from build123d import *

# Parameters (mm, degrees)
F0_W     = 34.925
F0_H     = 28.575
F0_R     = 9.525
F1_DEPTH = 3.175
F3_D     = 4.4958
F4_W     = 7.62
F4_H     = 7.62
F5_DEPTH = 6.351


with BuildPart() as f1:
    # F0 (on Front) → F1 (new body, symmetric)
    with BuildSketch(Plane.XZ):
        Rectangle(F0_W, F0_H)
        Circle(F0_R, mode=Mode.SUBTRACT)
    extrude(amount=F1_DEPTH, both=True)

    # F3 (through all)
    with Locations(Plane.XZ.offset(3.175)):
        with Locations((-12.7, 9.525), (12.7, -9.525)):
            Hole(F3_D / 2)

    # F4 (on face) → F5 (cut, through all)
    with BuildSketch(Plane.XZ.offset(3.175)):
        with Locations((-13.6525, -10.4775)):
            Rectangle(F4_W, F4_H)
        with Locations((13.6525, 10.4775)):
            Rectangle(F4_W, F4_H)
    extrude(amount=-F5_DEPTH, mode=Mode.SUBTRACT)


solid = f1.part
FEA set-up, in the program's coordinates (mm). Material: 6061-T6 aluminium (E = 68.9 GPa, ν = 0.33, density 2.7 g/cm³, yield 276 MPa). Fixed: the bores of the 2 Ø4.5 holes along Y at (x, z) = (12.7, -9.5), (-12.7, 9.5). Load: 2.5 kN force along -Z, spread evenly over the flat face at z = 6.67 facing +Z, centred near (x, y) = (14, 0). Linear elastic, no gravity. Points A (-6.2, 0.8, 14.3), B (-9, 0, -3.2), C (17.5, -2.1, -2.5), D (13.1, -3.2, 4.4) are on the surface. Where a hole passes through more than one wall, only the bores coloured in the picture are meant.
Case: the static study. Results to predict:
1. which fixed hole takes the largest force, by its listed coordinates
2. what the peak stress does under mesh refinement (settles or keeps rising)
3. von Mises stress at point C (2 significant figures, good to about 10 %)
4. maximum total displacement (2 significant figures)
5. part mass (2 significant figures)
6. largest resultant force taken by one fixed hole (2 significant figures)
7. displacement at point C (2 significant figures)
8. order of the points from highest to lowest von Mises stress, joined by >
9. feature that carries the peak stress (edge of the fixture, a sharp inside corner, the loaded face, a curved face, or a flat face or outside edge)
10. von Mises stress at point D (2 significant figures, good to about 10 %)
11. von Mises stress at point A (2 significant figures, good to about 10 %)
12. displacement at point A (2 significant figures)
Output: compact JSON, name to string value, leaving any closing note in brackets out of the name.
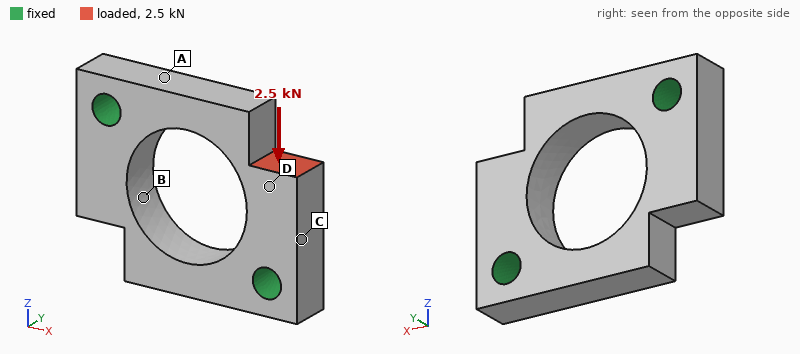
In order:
{"which fixed hole takes the largest force, by its listed coordinates": "(12.7, -9.5)", "what the peak stress does under mesh refinement": "keeps rising", "von Mises stress at point C": "42 MPa", "maximum total displacement": "11 µm", "part mass": "9.7 g", "largest resultant force taken by one fixed hole": "2.4 kN", "displacement at point C": "4.9 µm", "order of the points from highest to lowest von Mises stress, joined by >": "D > C > A > B", "feature that carries the peak stress": "edge of the fixture", "von Mises stress at point D": "54 MPa", "von Mises stress at point A": "14 MPa", "displacement at point A": "1.9 µm"}
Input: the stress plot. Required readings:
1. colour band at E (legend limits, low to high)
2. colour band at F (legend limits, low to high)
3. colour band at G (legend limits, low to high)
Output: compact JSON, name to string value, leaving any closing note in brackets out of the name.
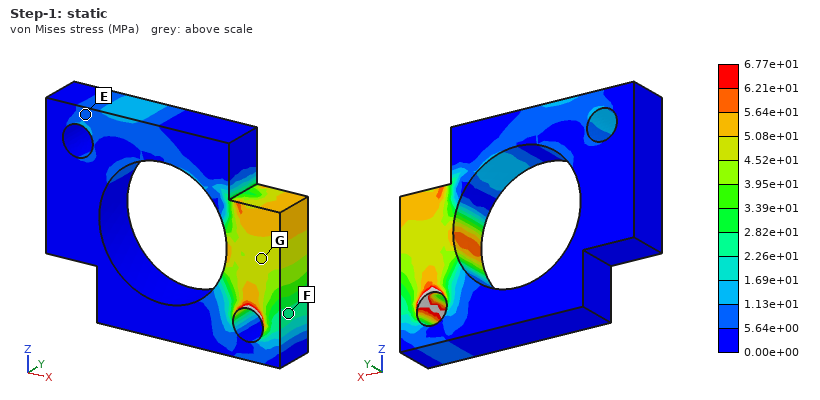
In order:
{"colour band at E": "5.64e+00 to 1.13e+01 MPa", "colour band at F": "2.26e+01 to 2.82e+01 MPa", "colour band at G": "4.52e+01 to 5.08e+01 MPa"}
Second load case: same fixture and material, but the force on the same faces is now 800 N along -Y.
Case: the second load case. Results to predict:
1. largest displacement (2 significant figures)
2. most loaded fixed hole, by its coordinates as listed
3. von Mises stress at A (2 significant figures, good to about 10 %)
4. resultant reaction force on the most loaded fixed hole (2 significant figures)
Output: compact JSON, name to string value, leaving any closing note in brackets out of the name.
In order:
{"largest displacement": "61 µm", "most loaded fixed hole, by its coordinates as listed": "(12.7, -9.5)", "von Mises stress at A": "20 MPa", "resultant reaction force on the most loaded fixed hole": "630 N"}
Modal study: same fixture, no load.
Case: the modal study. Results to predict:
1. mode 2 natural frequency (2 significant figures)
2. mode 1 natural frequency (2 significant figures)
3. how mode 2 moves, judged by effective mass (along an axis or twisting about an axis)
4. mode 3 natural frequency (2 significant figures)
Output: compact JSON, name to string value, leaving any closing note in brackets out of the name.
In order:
{"mode 2 natural frequency": "17 kHz", "mode 1 natural frequency": "16 kHz", "how mode 2 moves, judged by effective mass": "along Y", "mode 3 natural frequency": "31 kHz"}
